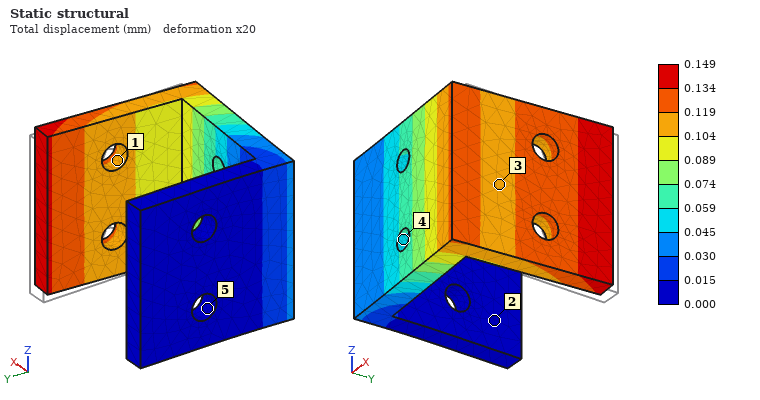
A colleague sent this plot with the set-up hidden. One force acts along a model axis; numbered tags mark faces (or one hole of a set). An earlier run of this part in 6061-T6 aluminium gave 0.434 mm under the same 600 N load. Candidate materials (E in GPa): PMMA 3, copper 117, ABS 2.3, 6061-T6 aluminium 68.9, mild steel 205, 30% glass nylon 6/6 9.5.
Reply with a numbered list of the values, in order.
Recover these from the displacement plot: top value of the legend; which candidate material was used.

1. 0.149 mm
2. mild steel
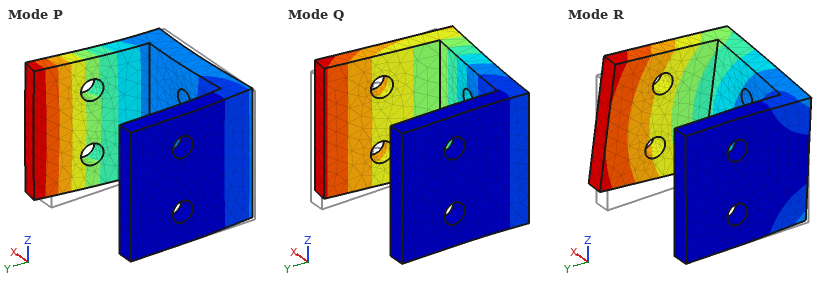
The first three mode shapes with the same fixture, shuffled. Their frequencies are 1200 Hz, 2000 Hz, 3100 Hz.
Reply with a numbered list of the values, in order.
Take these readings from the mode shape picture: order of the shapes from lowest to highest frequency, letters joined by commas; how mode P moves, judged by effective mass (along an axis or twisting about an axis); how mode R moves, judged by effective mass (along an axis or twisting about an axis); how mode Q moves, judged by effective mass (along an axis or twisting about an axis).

1. Q, R, P
2. along X
3. along Z
4. along Y
